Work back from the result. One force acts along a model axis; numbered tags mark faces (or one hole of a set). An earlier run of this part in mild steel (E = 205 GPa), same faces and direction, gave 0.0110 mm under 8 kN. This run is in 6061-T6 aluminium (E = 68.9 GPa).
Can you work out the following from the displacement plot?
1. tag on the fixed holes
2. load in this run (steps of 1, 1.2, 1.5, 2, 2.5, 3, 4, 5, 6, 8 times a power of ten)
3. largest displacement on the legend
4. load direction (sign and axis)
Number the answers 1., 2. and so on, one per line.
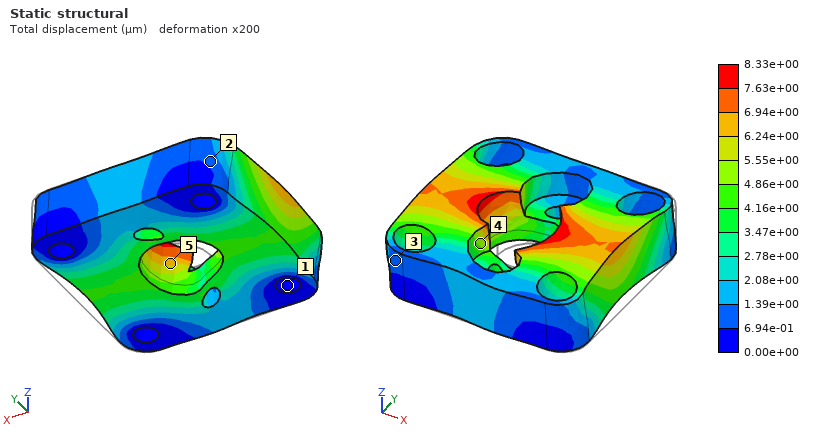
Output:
1. 1
2. 2 kN
3. 8.33e+00 µm
4. -X
